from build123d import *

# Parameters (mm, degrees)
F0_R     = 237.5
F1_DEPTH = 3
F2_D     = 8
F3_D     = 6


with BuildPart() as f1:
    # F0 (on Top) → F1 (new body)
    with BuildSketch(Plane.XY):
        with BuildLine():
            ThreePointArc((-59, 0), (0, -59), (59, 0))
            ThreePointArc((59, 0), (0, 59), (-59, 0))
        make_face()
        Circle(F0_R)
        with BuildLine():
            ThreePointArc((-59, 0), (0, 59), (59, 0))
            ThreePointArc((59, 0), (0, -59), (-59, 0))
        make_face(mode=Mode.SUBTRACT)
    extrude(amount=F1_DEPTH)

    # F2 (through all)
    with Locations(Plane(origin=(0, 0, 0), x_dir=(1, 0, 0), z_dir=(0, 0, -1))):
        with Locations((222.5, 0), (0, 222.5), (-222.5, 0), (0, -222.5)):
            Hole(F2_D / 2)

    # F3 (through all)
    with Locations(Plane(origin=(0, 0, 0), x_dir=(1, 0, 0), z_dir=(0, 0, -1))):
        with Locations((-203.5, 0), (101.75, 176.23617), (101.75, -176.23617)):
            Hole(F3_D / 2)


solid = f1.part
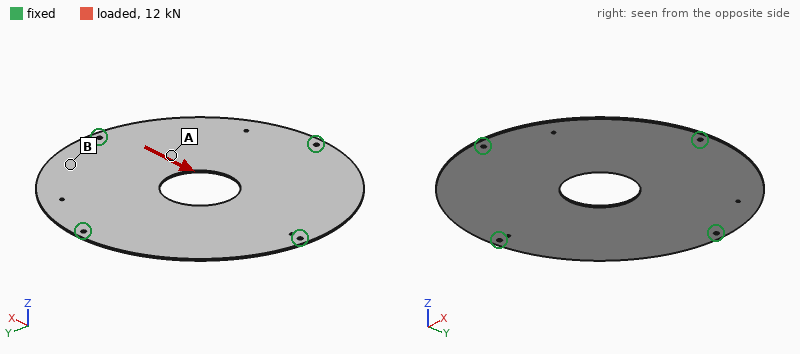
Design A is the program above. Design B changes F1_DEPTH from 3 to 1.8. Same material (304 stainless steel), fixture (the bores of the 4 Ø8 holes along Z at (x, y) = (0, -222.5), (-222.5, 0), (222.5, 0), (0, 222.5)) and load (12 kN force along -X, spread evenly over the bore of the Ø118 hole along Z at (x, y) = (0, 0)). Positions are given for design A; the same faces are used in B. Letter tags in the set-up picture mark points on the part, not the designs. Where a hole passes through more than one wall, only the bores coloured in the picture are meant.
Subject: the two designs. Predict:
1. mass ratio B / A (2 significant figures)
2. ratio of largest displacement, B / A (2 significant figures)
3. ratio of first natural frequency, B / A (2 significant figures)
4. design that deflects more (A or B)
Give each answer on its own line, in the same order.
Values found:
0.60
1.7
0.61
B
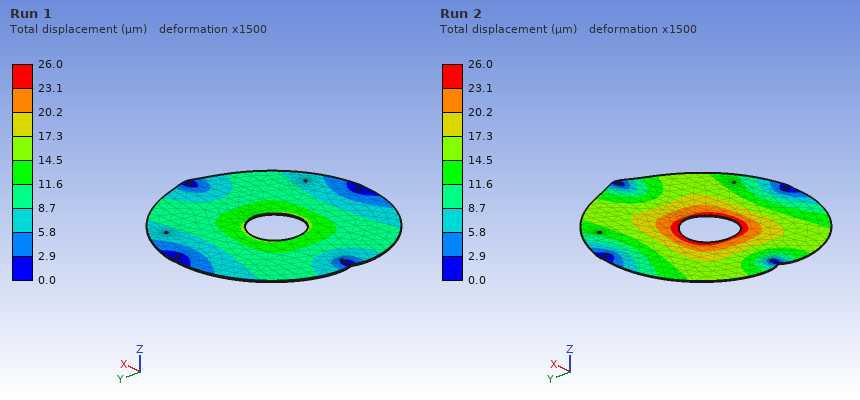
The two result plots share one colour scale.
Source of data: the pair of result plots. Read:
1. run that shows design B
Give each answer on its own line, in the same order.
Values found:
Run 2
